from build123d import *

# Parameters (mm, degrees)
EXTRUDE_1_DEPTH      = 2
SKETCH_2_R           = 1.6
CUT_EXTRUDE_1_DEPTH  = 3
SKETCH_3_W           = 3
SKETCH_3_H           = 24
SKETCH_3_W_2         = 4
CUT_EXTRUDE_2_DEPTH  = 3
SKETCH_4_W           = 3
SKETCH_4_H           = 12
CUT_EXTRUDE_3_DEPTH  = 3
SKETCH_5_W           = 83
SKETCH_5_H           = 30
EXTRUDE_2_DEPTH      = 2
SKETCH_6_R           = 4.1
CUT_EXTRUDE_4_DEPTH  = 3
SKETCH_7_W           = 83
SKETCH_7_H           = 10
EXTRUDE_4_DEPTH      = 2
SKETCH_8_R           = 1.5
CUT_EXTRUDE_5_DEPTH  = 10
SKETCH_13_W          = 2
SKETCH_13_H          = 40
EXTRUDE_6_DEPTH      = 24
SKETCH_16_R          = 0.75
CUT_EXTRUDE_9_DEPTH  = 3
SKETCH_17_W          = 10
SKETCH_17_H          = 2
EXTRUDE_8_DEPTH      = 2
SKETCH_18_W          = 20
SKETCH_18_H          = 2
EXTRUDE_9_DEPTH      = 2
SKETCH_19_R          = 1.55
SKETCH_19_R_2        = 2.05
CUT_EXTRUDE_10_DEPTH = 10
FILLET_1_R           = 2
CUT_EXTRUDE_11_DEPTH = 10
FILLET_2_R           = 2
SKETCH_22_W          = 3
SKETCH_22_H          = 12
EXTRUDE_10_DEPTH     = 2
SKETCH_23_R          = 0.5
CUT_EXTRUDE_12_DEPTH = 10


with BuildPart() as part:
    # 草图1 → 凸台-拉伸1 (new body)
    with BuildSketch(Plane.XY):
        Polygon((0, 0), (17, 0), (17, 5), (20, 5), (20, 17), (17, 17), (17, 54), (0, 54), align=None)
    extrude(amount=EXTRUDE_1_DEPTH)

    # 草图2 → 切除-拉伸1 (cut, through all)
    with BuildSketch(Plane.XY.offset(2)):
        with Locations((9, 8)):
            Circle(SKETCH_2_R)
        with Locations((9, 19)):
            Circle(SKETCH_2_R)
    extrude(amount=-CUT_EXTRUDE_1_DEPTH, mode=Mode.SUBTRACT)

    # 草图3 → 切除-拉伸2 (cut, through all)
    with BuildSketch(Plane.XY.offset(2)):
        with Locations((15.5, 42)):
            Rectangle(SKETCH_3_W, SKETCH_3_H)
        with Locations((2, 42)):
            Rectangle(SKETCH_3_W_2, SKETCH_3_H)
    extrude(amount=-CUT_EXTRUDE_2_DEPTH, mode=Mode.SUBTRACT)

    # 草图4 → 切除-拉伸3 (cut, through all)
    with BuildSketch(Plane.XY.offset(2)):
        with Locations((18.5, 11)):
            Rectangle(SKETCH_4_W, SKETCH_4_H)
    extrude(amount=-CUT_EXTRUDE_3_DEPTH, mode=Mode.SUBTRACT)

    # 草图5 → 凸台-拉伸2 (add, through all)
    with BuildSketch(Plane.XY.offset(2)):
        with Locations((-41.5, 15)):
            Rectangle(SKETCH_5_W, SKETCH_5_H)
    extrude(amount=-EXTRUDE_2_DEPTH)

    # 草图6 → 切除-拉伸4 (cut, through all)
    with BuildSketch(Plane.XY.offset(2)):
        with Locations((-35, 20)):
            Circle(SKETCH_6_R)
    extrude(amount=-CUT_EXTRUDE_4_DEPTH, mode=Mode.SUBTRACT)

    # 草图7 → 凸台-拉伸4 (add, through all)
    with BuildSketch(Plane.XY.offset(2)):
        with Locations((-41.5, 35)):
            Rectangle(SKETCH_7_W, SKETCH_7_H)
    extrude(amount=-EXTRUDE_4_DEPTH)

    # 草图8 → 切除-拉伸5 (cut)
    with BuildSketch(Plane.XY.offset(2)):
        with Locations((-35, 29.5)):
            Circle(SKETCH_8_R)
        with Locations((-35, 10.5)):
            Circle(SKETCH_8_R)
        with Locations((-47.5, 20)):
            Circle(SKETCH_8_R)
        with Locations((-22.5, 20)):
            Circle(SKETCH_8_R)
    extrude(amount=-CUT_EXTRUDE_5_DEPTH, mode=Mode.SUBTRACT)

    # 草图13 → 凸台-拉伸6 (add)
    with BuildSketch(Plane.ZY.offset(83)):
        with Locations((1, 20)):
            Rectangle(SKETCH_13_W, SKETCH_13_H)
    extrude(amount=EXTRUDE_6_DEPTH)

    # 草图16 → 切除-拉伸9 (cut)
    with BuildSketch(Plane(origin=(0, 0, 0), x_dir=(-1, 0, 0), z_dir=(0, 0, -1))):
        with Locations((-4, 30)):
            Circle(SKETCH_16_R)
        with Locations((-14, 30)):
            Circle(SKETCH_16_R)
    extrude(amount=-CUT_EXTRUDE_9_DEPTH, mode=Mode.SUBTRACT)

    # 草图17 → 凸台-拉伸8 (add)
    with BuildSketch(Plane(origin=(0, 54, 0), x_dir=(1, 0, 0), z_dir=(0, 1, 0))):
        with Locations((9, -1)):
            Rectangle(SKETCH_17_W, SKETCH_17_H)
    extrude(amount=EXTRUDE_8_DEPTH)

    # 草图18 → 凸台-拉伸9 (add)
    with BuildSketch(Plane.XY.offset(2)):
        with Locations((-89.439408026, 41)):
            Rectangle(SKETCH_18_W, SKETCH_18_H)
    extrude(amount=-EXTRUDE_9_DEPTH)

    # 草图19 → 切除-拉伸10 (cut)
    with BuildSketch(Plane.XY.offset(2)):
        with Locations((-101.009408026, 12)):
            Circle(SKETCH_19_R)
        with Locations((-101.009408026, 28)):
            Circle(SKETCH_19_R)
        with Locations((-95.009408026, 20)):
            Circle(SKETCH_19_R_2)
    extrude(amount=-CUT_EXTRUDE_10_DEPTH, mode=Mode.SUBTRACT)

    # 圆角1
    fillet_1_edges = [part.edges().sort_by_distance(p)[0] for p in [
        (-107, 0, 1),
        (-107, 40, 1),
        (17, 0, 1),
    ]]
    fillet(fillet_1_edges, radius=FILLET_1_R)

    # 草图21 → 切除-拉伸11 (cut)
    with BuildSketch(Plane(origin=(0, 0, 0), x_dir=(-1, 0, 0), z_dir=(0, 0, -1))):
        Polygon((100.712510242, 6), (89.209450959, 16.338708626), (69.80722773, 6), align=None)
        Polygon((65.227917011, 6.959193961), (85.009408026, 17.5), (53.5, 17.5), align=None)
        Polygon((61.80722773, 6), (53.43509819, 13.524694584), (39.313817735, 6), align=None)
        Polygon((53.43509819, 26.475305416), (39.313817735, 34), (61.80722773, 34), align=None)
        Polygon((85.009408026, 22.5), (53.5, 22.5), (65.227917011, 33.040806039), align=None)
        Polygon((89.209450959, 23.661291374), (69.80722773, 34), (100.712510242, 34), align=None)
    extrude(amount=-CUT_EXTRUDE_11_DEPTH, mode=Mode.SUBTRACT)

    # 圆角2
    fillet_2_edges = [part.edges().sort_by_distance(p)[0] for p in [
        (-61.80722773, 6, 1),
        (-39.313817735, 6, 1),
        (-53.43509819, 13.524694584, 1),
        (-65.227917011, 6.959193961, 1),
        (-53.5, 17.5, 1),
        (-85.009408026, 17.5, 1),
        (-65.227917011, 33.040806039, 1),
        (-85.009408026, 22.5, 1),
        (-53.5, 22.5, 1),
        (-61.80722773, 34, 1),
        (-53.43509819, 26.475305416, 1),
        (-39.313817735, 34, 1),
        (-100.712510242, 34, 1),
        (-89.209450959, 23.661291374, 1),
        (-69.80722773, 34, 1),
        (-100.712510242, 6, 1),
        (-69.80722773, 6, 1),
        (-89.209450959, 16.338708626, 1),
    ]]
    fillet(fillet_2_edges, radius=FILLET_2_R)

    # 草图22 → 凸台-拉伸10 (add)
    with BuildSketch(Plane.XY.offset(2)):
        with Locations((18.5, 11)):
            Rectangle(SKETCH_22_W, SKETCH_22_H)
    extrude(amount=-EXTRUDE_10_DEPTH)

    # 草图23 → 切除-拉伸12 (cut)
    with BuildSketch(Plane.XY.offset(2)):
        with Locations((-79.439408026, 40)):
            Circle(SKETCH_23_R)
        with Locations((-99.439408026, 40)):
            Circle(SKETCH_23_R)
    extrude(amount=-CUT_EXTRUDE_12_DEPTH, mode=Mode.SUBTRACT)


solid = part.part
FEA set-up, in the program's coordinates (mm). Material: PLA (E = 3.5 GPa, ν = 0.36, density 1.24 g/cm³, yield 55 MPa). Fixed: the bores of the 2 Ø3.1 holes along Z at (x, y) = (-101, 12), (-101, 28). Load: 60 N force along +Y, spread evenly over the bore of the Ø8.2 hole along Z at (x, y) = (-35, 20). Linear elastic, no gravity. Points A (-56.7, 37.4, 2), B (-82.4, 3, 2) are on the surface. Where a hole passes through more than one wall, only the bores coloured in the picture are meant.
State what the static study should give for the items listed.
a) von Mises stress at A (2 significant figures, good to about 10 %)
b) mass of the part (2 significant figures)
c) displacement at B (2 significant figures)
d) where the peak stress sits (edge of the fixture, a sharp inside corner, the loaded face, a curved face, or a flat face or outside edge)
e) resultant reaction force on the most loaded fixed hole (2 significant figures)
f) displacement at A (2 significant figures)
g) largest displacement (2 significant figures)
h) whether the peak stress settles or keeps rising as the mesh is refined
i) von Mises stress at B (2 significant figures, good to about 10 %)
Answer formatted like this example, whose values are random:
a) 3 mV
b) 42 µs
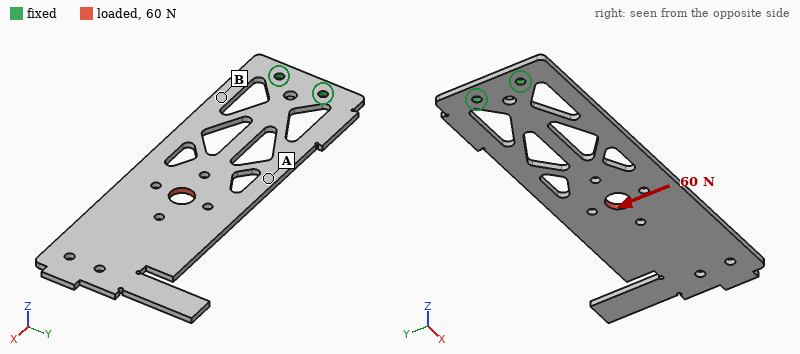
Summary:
a) 2.6 MPa
b) 11 g
c) 0.21 mm
d) edge of the fixture
e) 210 N
f) 0.47 mm
g) 1.3 mm
h) keeps rising
i) 7.3 MPa
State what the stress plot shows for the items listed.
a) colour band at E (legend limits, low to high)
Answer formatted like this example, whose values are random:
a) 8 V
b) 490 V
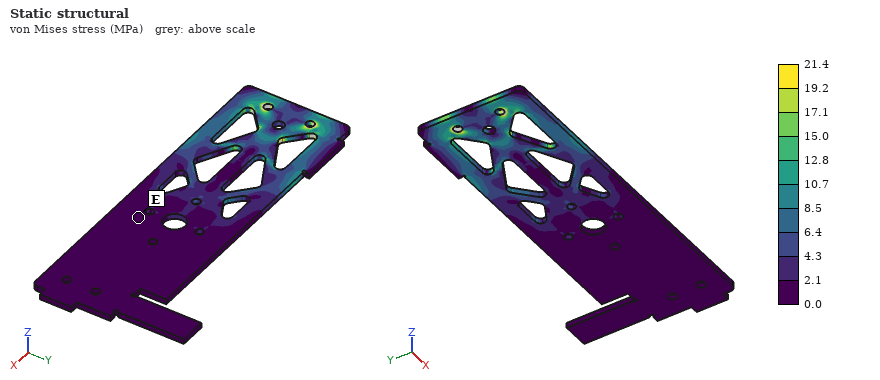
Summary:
a) 0.0 to 2.1 MPa
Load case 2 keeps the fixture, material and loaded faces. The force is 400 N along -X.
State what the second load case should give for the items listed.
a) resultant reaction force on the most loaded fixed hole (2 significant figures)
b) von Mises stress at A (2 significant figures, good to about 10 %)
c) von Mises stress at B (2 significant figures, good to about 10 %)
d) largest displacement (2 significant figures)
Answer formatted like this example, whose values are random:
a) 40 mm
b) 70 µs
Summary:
a) 210 N
b) 8.2 MPa
c) 7.1 MPa
d) 0.24 mm
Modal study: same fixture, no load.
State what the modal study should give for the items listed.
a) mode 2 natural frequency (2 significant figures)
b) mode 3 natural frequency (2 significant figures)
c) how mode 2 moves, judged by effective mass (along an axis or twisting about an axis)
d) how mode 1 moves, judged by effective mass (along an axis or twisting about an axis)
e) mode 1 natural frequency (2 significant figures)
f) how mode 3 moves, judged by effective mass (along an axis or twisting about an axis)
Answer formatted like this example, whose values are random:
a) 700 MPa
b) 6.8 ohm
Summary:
a) 150 Hz
b) 220 Hz
c) twisting about X
d) along Z
e) 29 Hz
f) along Z
